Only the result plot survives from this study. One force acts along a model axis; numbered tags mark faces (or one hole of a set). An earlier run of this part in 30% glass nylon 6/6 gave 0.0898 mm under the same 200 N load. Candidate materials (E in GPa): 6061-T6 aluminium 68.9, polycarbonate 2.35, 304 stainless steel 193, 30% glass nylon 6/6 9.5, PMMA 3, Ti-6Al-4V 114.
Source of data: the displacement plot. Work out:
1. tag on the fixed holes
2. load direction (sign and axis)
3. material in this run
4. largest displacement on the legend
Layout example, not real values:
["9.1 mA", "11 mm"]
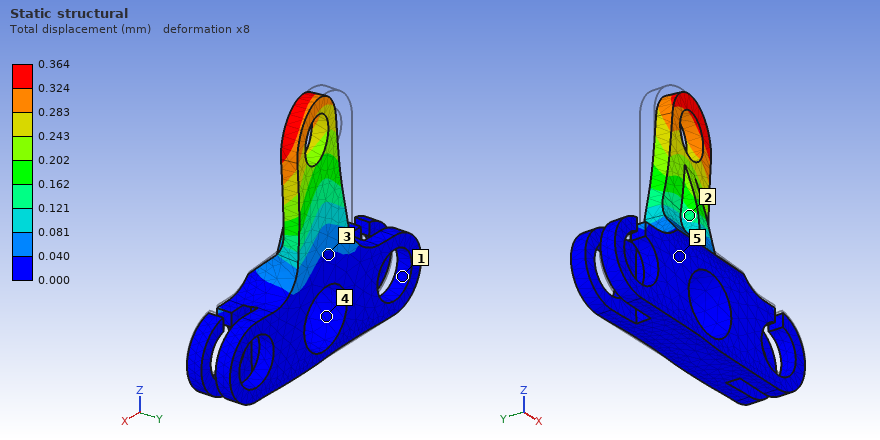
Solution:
["1", "+X", "polycarbonate", "0.364 mm"]
